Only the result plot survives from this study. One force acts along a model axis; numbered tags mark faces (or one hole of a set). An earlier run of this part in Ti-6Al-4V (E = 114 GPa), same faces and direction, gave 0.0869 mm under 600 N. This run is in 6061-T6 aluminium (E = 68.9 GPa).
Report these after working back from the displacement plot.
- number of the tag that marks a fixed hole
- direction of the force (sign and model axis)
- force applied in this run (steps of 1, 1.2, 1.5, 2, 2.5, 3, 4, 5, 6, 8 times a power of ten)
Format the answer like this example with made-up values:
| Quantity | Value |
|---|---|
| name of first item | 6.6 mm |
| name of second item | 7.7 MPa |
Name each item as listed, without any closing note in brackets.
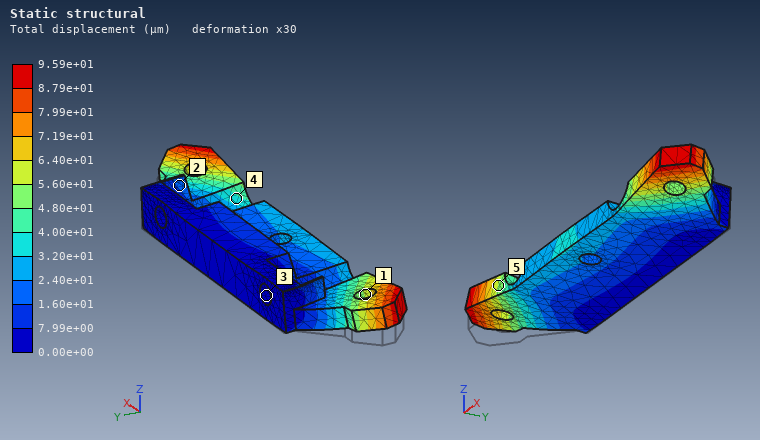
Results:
| Quantity | Value |
|---|---|
| number of the tag that marks a fixed hole | 3 |
| direction of the force | +Z |
| force applied in this run | 400 N |
